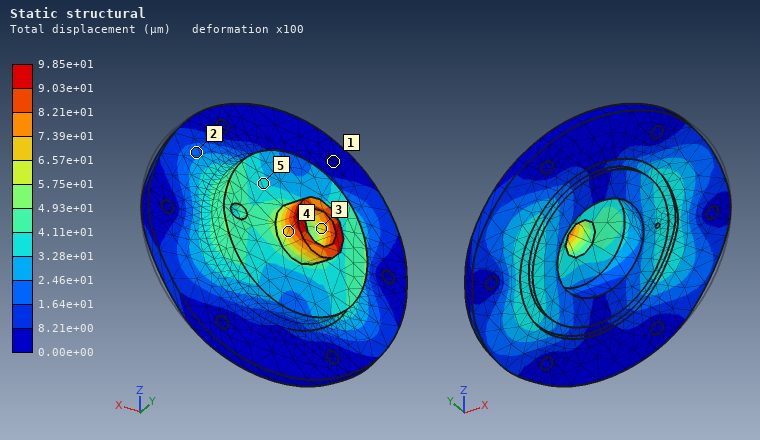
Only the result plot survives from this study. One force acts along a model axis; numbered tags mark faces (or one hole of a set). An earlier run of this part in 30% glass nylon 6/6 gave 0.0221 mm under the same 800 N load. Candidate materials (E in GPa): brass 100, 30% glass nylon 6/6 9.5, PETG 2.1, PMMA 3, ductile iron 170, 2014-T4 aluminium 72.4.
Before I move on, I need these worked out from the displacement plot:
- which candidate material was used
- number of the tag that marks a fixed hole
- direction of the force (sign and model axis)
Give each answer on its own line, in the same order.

PETG
1
-X
